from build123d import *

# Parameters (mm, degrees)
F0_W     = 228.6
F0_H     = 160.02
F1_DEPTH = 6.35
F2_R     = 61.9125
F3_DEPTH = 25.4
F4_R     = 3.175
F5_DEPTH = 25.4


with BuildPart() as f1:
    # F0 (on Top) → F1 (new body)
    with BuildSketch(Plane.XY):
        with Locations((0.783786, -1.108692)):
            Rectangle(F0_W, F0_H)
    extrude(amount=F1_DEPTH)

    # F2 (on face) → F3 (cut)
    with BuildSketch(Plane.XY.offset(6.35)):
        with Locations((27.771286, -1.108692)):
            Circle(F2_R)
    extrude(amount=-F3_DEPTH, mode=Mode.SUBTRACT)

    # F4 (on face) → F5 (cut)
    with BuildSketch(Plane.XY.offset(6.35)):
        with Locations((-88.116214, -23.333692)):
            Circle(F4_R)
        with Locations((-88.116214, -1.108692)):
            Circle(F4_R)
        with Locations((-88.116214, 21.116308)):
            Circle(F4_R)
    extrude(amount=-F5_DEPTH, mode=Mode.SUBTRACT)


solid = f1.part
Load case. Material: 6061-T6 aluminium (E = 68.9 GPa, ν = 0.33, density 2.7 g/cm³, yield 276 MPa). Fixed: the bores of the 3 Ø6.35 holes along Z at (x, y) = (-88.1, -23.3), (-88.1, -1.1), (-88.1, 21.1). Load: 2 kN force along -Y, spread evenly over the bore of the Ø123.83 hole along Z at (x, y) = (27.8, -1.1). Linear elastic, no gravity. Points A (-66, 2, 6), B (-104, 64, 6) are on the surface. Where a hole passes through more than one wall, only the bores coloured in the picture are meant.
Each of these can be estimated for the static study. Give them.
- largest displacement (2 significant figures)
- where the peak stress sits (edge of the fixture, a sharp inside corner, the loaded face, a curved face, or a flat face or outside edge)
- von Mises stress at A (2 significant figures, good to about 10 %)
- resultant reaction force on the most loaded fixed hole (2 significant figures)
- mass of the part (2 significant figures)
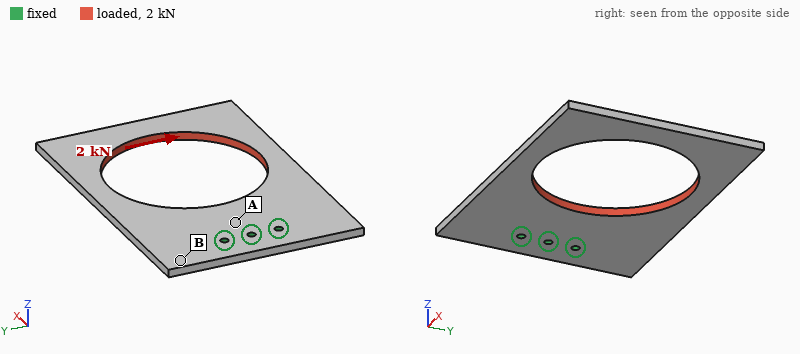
0.25 mm
edge of the fixture
22 MPa
4.7 kN
420 g
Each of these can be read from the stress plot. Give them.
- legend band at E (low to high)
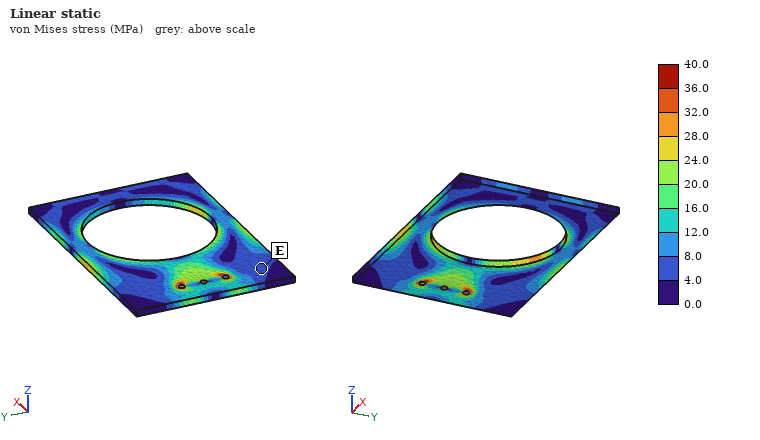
4.0 to 8.0 MPa
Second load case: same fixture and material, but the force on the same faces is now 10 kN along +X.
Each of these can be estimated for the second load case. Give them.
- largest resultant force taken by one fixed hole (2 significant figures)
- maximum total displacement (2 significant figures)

4.8 kN
0.16 mm
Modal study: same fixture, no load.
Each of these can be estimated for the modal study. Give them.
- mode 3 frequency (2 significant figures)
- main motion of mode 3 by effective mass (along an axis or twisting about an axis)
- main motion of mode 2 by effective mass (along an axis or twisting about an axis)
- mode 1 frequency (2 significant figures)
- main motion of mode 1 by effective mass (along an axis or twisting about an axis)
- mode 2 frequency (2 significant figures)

640 Hz
along Z
twisting about X
110 Hz
along Z
270 Hz
